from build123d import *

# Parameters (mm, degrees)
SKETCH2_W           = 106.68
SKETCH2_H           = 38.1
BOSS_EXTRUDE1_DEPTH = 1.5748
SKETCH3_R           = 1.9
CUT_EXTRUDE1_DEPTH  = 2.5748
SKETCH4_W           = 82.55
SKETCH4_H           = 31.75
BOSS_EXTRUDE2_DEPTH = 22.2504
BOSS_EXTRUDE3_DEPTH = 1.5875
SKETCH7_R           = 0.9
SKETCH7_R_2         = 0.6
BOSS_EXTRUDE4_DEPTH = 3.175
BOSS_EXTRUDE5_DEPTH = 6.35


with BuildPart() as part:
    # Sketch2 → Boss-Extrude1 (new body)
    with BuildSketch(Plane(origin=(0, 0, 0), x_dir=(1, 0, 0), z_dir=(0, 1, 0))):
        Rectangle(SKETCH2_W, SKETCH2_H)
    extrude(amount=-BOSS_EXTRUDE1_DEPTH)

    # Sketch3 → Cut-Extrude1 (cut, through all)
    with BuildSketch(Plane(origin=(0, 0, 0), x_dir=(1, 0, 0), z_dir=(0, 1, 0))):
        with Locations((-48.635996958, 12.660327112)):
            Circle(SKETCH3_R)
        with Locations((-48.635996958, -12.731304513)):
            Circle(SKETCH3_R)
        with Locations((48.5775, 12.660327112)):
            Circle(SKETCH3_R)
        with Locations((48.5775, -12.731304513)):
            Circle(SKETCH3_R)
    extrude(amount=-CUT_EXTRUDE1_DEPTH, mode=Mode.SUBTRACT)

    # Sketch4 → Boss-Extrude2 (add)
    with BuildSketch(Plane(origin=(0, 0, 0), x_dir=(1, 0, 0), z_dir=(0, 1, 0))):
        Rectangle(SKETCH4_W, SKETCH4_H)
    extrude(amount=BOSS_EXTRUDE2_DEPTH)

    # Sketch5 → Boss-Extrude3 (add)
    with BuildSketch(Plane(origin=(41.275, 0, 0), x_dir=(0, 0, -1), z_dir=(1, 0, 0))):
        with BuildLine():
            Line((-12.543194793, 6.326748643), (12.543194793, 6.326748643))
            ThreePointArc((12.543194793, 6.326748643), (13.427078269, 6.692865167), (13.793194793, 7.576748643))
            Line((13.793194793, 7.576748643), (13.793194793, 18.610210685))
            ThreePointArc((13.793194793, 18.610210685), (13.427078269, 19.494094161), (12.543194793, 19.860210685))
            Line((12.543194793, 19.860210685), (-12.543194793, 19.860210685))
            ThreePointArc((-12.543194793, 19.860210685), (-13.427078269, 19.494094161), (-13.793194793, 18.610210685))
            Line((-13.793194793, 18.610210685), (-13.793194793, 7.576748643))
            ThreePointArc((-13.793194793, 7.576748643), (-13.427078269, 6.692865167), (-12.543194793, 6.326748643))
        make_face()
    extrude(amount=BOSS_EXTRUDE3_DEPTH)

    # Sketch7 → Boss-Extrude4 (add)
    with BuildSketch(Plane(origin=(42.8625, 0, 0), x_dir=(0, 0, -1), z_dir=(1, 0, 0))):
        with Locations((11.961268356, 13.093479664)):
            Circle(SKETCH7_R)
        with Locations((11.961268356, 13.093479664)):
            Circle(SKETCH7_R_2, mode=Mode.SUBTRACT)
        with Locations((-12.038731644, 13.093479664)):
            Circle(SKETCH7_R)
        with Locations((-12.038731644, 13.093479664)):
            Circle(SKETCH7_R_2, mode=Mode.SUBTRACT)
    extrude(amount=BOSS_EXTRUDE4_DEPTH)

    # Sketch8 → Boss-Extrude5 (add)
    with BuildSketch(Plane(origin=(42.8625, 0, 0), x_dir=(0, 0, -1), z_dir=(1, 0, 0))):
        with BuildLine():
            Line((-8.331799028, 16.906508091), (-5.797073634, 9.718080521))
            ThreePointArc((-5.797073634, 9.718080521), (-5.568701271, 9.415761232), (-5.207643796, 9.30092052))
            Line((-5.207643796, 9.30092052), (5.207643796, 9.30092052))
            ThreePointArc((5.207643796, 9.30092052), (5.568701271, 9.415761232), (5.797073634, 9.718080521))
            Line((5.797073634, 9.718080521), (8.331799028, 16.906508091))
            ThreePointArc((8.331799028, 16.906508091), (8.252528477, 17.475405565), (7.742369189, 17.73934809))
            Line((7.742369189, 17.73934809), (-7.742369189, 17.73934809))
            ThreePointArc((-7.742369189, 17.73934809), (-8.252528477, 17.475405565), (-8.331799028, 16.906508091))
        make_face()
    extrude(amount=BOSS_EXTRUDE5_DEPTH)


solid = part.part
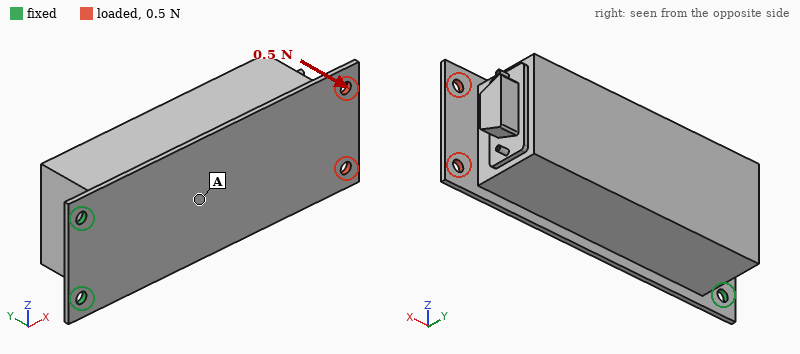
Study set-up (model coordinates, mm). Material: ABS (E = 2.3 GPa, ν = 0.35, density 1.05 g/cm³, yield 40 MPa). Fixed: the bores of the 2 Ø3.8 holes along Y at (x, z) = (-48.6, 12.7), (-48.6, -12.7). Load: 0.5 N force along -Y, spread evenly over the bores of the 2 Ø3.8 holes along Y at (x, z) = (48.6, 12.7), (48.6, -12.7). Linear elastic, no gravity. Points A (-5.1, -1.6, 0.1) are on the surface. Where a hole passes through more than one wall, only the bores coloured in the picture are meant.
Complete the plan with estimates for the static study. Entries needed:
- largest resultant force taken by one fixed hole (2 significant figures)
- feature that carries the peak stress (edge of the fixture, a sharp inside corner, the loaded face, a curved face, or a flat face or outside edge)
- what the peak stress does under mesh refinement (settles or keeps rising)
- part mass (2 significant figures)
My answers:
0.30 N
edge of the fixture
keeps rising
69 g
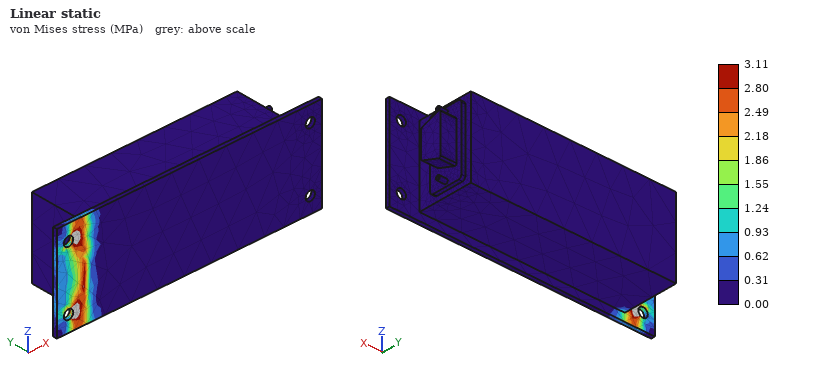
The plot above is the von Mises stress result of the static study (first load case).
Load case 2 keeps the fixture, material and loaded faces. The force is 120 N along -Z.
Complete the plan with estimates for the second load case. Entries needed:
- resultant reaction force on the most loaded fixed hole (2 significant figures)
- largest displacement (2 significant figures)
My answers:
440 N
1.4 mm
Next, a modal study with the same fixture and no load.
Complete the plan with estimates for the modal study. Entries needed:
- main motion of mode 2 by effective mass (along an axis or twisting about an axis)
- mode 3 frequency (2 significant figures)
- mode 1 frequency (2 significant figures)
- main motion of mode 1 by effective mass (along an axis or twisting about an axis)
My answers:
along Z
500 Hz
22 Hz
along Y
